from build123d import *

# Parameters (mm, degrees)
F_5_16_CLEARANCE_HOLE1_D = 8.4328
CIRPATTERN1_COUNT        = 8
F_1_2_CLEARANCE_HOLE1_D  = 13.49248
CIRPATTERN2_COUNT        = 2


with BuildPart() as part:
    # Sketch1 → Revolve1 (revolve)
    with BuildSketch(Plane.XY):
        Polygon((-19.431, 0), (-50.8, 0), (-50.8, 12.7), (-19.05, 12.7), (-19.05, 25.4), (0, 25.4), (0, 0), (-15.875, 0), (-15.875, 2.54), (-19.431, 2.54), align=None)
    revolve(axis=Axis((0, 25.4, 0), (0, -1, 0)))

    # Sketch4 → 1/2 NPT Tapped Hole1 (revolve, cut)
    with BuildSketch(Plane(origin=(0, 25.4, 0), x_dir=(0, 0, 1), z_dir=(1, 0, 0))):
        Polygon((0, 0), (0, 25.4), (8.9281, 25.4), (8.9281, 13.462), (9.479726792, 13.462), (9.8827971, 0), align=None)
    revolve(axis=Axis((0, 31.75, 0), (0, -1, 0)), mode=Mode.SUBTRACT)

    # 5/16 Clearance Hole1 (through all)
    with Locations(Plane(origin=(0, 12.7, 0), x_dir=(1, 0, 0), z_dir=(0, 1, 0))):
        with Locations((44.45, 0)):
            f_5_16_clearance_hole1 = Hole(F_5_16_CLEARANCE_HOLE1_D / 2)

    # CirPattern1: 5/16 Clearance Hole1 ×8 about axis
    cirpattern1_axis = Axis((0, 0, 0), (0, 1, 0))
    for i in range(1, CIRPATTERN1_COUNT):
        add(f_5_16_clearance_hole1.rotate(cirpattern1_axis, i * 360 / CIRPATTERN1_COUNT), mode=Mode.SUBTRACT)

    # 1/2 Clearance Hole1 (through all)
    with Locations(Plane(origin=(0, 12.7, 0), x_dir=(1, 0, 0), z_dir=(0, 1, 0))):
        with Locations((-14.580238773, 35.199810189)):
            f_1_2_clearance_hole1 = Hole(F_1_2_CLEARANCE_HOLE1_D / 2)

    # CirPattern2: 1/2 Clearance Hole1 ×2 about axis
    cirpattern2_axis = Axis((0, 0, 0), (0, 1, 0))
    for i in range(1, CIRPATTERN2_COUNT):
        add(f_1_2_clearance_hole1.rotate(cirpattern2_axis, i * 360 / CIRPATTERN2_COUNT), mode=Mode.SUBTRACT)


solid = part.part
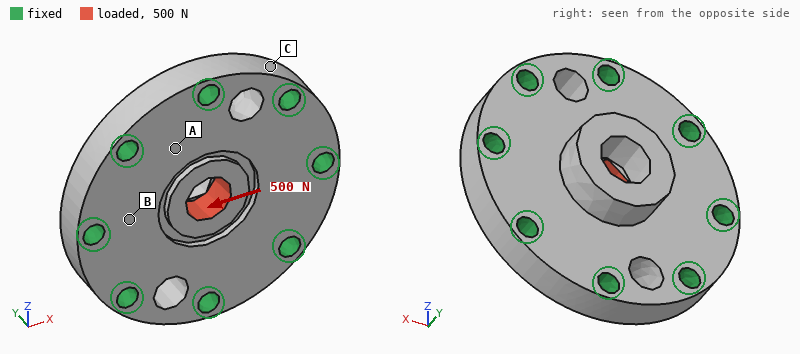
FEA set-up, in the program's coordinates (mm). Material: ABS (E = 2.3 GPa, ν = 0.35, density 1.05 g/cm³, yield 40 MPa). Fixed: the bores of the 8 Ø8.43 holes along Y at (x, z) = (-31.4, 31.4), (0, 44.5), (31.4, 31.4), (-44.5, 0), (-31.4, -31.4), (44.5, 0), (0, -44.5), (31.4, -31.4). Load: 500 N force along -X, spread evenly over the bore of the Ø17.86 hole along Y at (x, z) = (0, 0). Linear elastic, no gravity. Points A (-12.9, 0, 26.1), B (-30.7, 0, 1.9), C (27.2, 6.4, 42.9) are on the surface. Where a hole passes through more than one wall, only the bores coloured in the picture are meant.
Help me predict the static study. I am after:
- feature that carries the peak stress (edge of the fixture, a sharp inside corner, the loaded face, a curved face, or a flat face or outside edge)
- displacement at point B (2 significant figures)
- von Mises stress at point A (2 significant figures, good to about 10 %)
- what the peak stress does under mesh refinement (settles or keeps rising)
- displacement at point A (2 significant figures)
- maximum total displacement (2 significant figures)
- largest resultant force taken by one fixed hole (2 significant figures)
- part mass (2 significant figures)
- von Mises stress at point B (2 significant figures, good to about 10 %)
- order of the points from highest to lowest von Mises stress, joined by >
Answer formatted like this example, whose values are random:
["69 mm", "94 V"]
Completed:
["a sharp inside corner", "1.9 µm", "0.23 MPa", "keeps rising", "1.6 µm", "9.9 µm", "110 N", "110 g", "0.40 MPa", "B > A > C"]
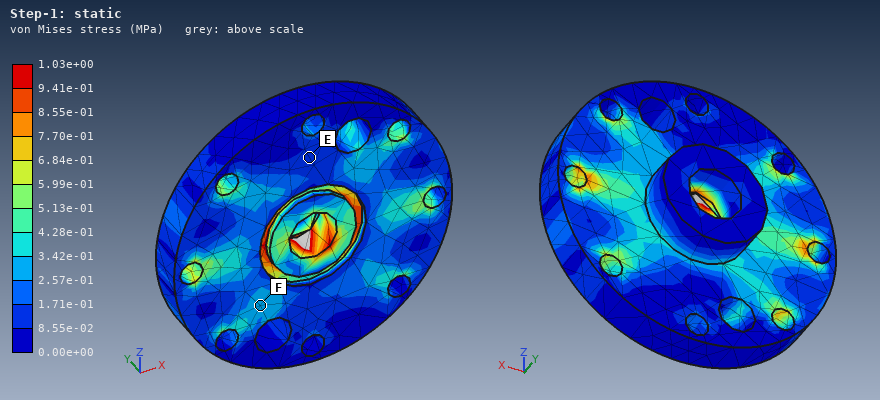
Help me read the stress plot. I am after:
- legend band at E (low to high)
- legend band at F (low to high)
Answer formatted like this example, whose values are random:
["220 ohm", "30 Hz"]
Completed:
["8.55e-02 to 1.71e-01 MPa", "2.57e-01 to 3.42e-01 MPa"]
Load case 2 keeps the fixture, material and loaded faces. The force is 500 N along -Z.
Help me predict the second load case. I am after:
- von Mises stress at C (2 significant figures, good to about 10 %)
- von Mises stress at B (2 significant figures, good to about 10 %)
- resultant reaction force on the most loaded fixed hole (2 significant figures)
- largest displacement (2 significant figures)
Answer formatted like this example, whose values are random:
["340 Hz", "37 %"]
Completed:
["0.078 MPa", "0.11 MPa", "110 N", "10.0 µm"]
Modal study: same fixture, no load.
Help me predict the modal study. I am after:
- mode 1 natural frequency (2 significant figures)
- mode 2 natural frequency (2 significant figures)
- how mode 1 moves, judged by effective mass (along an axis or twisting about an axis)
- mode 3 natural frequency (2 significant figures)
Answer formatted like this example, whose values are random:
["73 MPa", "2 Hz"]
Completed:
["3600 Hz", "5500 Hz", "along Y", "5500 Hz"]
